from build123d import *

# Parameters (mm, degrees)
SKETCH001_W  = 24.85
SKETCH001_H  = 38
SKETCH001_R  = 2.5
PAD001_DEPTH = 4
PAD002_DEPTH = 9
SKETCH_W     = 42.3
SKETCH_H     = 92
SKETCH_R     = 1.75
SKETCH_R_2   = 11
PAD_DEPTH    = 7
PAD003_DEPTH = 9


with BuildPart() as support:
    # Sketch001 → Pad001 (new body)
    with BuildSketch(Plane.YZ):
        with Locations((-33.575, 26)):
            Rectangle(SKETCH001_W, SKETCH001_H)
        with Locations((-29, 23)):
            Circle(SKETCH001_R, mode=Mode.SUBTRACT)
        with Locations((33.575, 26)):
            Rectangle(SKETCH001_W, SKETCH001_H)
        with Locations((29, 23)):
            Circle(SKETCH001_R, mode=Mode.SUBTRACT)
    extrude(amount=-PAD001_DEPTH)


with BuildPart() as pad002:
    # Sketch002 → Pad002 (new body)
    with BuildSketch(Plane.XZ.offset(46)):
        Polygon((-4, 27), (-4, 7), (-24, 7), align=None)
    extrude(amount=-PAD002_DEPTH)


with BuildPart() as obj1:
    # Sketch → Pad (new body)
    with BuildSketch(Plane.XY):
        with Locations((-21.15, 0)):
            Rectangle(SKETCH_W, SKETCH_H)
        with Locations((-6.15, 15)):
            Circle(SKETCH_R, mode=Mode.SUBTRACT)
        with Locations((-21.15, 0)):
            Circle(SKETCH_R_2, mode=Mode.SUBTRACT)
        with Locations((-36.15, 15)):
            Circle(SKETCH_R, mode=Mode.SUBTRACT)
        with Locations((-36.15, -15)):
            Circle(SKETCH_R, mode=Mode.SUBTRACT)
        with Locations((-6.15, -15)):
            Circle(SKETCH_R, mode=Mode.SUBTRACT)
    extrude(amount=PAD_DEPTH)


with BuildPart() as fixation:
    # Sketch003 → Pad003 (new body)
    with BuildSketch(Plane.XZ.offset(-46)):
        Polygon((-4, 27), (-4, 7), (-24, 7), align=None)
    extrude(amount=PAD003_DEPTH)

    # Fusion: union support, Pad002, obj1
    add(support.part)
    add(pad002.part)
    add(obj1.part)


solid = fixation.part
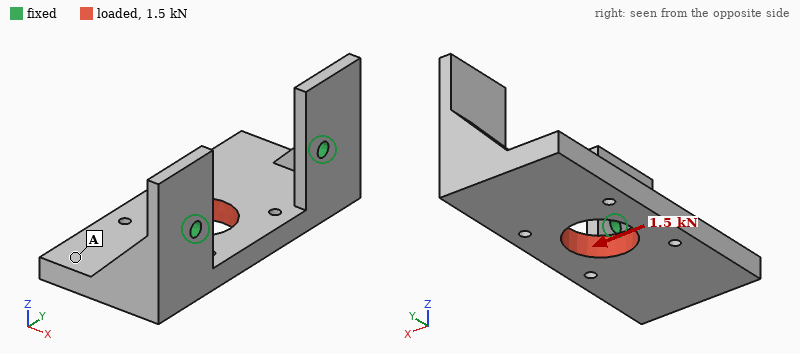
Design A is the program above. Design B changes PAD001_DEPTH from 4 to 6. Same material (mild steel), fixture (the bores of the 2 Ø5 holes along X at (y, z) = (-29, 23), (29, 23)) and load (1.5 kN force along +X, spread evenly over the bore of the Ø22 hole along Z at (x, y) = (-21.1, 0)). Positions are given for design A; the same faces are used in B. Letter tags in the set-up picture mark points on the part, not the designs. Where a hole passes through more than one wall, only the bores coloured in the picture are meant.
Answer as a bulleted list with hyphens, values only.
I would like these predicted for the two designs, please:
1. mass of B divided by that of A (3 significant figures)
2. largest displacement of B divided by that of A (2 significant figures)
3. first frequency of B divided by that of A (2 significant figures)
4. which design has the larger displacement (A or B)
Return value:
- 1.09
- 0.43
- 1.5
- A
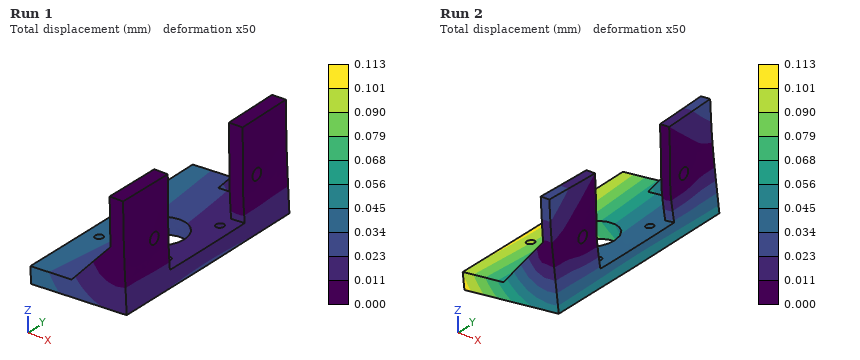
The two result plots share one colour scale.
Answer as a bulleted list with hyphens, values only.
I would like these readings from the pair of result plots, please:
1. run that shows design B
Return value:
- Run 1
